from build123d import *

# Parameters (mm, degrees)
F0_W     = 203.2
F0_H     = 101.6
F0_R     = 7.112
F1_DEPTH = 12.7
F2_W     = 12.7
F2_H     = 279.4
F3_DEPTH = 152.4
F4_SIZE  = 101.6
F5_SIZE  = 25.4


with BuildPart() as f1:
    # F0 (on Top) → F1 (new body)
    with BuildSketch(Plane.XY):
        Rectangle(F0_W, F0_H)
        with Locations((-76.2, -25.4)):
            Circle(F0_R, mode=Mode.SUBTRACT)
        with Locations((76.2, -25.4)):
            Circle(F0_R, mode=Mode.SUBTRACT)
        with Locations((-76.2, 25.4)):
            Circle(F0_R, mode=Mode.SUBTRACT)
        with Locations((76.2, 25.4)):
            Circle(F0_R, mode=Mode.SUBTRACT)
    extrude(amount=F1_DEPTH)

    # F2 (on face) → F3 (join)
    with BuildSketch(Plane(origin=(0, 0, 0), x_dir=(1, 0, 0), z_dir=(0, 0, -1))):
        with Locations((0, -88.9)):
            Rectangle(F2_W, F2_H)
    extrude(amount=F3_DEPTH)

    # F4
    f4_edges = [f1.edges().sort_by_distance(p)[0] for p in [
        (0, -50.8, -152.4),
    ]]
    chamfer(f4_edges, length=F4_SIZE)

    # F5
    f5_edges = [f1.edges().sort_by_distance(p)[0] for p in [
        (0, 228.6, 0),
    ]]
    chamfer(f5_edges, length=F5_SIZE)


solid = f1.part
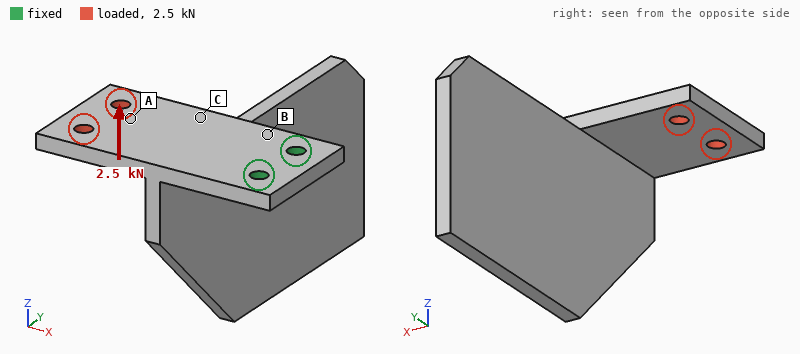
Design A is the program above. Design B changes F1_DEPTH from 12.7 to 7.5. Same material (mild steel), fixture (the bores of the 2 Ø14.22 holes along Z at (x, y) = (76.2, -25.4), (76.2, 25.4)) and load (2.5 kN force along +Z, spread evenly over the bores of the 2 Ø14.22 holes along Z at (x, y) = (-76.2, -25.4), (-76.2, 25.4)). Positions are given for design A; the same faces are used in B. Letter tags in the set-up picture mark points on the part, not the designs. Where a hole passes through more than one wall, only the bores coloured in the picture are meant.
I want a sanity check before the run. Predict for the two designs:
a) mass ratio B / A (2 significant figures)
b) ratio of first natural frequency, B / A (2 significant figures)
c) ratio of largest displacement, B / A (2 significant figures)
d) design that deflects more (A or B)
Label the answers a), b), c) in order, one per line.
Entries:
a) 0.86
b) 0.59
c) 4.6
d) B
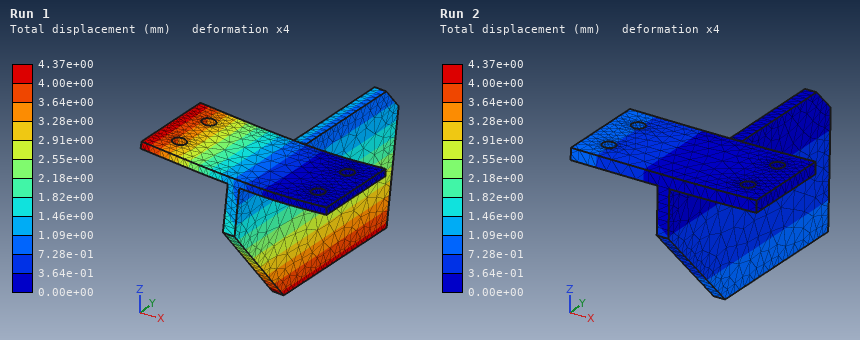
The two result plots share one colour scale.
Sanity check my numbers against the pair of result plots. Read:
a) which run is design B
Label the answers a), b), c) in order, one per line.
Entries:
a) Run 1
